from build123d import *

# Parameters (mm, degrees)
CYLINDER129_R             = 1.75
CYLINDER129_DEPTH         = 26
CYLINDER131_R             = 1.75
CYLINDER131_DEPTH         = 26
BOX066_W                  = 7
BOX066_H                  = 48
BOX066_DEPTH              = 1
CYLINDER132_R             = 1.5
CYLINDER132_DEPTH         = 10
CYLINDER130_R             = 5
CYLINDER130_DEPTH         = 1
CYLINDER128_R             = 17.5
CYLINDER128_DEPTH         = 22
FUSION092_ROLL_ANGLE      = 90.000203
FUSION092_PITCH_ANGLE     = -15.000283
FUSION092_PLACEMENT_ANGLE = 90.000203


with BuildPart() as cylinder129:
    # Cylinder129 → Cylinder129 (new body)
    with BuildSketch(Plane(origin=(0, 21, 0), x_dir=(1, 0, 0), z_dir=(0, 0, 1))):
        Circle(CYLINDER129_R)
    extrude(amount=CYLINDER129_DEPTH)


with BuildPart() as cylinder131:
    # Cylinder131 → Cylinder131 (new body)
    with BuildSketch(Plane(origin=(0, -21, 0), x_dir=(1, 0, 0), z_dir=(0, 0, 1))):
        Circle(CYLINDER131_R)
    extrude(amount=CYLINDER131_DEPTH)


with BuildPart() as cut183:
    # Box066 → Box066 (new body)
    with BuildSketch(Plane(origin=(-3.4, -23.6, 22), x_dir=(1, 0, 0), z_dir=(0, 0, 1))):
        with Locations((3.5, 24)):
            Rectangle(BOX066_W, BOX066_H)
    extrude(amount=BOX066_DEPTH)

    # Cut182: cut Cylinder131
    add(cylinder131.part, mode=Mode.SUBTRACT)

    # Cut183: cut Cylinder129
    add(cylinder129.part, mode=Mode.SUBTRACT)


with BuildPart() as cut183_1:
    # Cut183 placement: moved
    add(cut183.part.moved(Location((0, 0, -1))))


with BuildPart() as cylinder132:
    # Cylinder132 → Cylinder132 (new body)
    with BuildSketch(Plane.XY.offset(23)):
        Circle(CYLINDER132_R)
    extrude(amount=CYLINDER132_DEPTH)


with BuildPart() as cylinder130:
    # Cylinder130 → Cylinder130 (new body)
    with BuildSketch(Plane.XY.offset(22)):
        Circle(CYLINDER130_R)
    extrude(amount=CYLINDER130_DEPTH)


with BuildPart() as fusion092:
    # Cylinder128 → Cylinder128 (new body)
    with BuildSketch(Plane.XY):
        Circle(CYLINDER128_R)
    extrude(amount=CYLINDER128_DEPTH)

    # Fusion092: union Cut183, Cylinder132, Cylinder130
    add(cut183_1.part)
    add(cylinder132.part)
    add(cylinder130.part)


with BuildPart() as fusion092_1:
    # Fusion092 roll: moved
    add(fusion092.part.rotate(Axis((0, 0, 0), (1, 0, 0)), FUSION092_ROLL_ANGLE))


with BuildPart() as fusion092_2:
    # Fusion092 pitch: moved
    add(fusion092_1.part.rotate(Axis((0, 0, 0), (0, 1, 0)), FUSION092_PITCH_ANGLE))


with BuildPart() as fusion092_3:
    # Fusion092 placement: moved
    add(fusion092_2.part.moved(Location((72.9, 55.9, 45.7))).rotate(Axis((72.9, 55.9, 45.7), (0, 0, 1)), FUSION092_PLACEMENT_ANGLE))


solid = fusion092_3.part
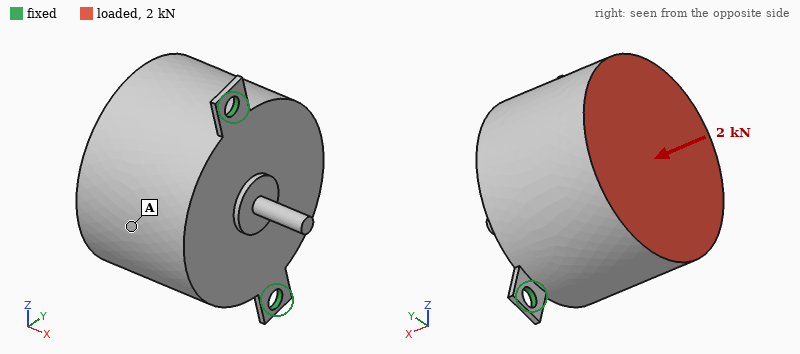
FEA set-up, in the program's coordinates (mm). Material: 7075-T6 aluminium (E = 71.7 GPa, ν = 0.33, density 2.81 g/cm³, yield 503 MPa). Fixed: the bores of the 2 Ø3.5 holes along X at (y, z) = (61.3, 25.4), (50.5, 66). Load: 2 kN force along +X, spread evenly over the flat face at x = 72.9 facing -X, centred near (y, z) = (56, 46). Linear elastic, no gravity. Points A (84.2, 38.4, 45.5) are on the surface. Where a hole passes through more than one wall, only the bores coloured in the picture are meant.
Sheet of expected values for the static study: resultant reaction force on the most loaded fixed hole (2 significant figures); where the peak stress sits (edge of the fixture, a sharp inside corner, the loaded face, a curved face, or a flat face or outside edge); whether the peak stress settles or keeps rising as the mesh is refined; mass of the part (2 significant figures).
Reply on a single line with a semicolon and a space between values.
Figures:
1.2 kN; edge of the fixture; keeps rising; 60 g
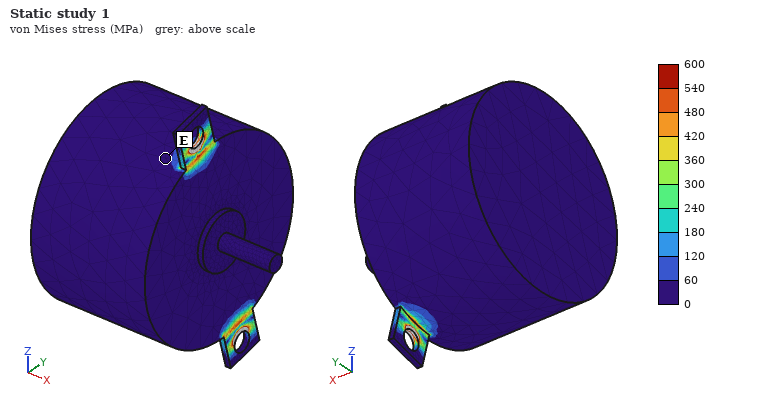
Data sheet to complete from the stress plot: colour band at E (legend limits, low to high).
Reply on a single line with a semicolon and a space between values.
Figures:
0 to 60 MPa
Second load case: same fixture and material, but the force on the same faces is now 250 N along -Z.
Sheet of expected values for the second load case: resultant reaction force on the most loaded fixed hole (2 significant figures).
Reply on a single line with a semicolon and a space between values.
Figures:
190 N
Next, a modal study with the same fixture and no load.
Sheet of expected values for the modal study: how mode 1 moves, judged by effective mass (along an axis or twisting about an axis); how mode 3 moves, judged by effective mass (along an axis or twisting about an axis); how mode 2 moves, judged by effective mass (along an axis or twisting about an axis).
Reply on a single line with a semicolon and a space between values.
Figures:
along Y; along Z; along X
